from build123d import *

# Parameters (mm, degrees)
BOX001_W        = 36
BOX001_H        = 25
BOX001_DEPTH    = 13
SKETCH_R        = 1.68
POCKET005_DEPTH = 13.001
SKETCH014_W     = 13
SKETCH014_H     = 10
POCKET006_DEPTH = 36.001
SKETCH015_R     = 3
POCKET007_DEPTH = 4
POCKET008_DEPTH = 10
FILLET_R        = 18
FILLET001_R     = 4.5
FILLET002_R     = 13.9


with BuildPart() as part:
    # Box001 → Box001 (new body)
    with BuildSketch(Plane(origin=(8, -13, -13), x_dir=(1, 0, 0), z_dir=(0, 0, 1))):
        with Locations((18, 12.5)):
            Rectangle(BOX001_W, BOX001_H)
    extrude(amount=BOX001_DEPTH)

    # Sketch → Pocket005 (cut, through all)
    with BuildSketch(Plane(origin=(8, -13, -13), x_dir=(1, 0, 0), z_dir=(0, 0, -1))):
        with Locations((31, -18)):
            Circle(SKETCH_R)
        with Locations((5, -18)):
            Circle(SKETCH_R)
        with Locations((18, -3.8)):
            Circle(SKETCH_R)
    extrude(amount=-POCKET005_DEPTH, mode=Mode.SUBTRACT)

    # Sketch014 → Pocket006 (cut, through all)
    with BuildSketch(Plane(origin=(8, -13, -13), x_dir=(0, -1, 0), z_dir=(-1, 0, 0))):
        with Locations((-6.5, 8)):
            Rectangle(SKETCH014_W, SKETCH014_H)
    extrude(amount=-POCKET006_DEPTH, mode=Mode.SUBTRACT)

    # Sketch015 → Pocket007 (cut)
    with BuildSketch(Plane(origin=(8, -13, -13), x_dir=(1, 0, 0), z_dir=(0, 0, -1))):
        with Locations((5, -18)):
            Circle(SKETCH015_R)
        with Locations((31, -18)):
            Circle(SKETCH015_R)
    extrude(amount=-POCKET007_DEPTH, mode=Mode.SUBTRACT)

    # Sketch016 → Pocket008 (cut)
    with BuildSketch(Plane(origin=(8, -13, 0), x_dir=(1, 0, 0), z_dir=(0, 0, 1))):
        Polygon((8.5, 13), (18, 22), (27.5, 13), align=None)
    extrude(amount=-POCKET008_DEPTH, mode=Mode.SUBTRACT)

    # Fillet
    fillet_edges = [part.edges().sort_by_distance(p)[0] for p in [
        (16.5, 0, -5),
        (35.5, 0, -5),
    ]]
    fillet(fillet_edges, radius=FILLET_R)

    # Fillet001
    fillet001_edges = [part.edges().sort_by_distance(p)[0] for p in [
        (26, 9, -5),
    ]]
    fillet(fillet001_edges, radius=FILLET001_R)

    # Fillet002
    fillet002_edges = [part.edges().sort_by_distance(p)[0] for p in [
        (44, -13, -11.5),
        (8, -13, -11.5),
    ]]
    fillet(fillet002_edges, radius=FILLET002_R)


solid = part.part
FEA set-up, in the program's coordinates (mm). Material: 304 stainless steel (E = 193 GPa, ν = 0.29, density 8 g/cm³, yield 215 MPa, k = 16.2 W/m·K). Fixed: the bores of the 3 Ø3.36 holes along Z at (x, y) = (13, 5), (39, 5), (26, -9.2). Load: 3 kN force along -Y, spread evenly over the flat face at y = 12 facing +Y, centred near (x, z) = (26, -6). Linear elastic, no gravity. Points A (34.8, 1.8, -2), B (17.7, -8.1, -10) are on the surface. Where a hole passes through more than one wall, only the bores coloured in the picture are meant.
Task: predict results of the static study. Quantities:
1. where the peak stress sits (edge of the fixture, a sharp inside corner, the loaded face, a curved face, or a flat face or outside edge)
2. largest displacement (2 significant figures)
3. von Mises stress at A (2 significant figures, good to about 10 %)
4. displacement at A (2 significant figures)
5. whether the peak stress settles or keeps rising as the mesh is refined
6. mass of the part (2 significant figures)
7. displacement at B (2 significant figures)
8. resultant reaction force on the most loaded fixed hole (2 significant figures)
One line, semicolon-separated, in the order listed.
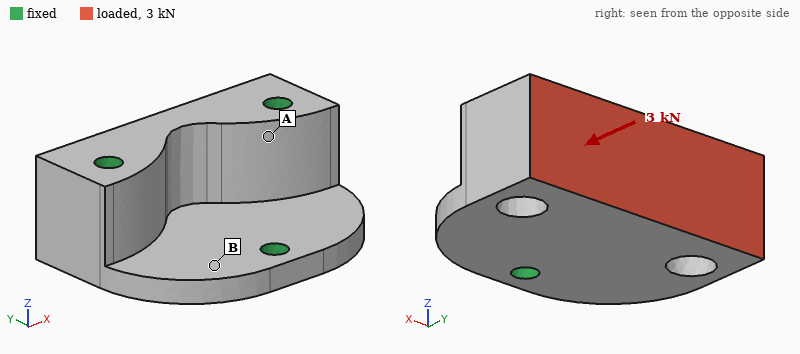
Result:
edge of the fixture; 1.5 µm; 9.9 MPa; 0.53 µm; keeps rising; 43 g; 0.49 µm; 1.3 kN
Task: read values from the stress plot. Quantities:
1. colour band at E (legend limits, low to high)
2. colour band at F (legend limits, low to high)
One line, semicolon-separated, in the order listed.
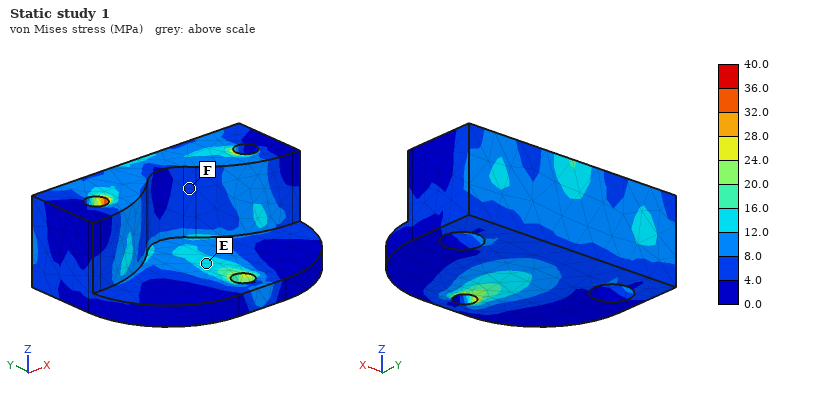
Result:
12.0 to 16.0 MPa; 4.0 to 8.0 MPa
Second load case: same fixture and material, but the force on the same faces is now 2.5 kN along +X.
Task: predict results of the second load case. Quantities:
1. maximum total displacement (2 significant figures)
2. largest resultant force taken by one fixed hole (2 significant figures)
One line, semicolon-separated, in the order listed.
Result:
1.7 µm; 1.4 kN
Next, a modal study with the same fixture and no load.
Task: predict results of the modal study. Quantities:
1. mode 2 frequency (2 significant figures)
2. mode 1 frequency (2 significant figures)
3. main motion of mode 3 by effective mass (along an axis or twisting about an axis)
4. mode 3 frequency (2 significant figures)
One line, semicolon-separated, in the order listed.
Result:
28 kHz; 27 kHz; along Z; 40 kHz
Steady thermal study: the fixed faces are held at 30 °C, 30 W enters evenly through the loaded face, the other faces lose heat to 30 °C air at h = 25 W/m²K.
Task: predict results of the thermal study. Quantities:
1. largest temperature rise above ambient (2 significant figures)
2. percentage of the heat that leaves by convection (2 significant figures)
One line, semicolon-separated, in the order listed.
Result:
58 K; 3.8 %
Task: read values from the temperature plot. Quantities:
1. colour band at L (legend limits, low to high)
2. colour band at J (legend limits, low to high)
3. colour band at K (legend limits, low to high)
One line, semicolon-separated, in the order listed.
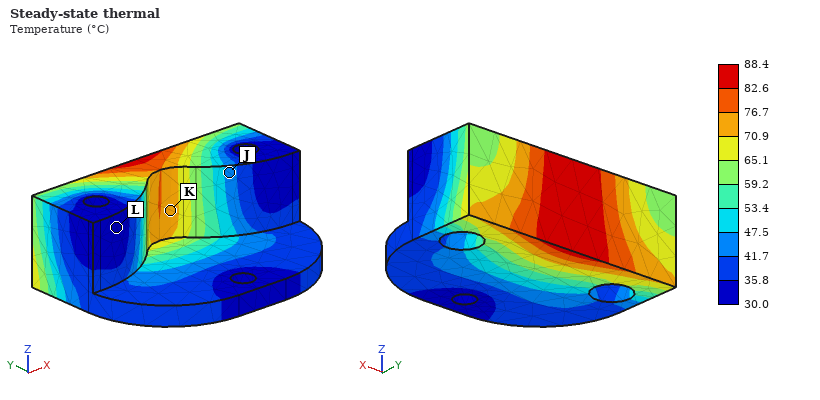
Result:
30.0 to 35.8 °C; 41.7 to 47.5 °C; 70.9 to 76.7 °C
